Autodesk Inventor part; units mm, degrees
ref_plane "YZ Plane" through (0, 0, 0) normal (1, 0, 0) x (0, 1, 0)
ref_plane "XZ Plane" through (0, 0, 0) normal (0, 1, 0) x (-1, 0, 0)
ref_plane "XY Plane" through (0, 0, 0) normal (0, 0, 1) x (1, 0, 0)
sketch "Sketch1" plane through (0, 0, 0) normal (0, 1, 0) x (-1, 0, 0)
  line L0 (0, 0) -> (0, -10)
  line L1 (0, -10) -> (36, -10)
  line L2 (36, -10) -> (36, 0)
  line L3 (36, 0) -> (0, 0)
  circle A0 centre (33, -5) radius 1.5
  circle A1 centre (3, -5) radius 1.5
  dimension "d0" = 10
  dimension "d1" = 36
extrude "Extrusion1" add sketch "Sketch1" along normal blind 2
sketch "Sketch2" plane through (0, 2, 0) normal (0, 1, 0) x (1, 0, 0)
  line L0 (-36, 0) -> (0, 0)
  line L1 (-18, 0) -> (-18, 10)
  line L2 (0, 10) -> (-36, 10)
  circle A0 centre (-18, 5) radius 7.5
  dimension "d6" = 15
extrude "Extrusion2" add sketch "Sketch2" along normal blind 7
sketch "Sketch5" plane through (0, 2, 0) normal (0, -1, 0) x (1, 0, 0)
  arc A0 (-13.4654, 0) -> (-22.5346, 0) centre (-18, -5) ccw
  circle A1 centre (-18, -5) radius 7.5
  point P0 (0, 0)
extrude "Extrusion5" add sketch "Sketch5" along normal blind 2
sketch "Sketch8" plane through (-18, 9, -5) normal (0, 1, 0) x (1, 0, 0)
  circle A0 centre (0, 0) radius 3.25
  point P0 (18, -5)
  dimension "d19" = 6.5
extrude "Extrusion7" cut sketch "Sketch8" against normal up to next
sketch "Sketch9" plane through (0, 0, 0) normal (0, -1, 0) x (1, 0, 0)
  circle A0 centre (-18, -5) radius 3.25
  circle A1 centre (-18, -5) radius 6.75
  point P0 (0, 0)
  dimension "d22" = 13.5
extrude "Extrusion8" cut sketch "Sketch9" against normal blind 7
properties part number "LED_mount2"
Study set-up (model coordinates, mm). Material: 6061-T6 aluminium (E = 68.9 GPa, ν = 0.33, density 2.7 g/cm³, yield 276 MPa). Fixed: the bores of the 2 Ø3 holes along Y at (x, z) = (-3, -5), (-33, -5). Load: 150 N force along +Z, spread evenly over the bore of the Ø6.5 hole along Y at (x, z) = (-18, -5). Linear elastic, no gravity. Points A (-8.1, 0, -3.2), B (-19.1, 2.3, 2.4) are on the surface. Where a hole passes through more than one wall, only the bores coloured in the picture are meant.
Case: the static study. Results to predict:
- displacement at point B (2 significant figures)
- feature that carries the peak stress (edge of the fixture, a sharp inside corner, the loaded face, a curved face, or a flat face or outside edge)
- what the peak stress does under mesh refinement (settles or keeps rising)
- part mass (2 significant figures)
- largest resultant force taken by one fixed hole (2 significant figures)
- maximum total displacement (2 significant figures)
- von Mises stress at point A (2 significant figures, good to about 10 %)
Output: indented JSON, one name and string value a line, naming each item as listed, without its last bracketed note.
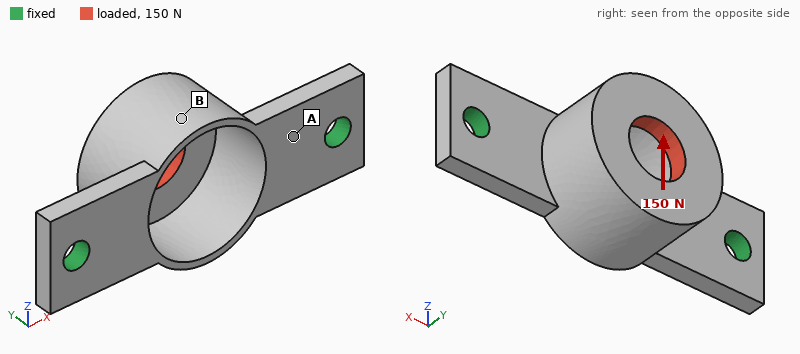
{
  "displacement at point B": "54 µm",
  "feature that carries the peak stress": "edge of the fixture",
  "what the peak stress does under mesh refinement": "keeps rising",
  "part mass": "2.5 g",
  "largest resultant force taken by one fixed hole": "75 N",
  "maximum total displacement": "82 µm",
  "von Mises stress at point A": "61 MPa"
}
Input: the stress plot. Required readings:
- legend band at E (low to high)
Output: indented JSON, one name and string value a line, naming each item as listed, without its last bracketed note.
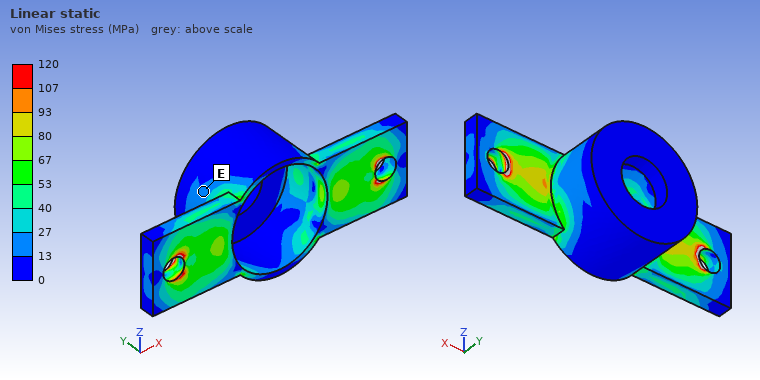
{
  "legend band at E": "13 to 27 MPa"
}
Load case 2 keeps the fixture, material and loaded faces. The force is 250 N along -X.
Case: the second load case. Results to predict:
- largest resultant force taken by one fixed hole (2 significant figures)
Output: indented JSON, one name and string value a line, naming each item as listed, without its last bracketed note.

{
  "largest resultant force taken by one fixed hole": "150 N"
}
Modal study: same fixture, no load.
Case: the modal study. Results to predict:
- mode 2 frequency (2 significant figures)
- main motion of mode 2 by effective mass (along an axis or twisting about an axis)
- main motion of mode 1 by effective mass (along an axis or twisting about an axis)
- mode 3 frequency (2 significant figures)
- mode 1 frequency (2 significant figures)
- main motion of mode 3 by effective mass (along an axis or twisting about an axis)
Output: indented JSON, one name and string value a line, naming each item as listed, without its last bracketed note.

{
  "mode 2 frequency": "12 kHz",
  "main motion of mode 2 by effective mass": "along Y",
  "main motion of mode 1 by effective mass": "along Z",
  "mode 3 frequency": "16 kHz",
  "mode 1 frequency": "6900 Hz",
  "main motion of mode 3 by effective mass": "along X"
}
